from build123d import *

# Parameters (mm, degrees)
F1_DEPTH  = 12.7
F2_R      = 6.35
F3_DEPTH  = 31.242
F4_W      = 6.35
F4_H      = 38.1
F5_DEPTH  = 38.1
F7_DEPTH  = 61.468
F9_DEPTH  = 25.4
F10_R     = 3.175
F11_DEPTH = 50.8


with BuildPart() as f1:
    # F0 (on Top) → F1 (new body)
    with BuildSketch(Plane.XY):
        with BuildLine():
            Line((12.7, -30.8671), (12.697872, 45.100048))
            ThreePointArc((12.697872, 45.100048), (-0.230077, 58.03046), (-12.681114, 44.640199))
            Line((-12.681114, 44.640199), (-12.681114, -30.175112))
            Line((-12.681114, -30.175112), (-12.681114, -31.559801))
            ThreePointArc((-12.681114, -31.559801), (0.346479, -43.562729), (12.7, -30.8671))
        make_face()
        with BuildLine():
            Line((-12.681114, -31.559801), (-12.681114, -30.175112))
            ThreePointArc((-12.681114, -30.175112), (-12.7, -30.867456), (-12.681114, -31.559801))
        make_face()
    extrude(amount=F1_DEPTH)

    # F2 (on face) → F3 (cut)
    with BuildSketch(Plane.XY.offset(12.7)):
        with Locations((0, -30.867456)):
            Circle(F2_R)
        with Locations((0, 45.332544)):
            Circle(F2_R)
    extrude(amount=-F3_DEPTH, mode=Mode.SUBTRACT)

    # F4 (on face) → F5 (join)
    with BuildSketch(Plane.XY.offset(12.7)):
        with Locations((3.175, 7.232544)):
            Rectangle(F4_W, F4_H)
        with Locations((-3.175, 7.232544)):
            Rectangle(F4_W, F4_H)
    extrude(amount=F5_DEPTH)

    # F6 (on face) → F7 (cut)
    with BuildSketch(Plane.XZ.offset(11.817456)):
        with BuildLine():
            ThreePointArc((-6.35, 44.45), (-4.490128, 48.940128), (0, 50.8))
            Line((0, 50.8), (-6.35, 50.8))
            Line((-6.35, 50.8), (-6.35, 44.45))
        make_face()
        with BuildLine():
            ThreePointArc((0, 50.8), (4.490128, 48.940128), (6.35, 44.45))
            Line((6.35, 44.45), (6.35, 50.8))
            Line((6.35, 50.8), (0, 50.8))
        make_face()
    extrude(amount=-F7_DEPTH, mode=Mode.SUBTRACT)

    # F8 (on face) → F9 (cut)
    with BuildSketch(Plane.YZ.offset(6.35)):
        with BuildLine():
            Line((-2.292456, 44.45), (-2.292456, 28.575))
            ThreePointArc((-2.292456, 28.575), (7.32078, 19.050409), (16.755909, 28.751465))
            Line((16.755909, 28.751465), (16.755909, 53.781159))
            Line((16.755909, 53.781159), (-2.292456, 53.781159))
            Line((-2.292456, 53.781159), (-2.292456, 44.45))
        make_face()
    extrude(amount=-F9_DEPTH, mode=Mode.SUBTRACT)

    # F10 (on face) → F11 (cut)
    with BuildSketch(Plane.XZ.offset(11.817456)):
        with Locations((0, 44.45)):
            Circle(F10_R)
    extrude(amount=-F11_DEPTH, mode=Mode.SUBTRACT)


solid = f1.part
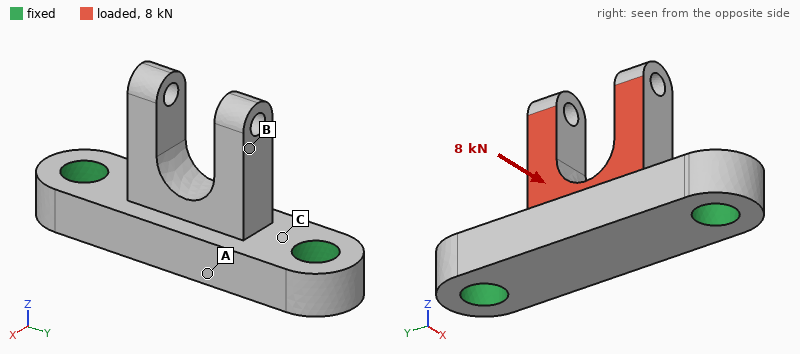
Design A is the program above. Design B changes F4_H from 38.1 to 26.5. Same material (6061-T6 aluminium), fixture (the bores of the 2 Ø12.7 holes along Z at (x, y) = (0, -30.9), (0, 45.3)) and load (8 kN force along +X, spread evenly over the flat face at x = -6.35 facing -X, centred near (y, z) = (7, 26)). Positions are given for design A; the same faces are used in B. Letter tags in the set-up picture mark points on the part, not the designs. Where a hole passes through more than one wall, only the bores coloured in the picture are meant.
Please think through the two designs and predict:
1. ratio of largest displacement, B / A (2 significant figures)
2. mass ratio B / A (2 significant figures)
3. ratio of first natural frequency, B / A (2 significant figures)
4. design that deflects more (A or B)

1.3
0.87
0.87
B
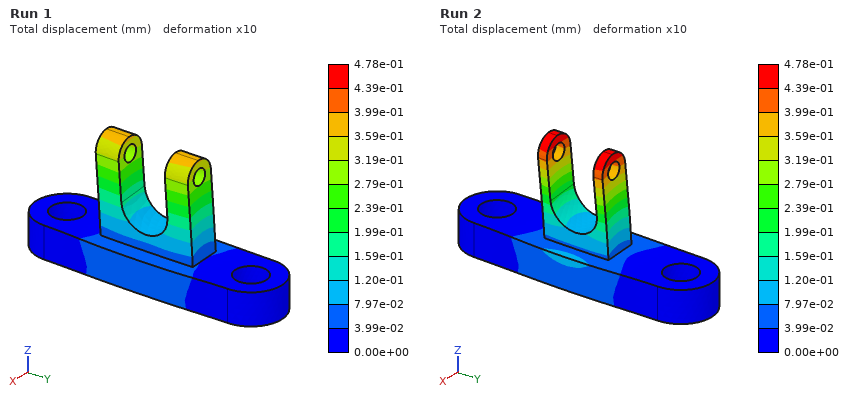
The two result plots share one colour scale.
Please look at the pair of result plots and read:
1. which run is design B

Run 2
